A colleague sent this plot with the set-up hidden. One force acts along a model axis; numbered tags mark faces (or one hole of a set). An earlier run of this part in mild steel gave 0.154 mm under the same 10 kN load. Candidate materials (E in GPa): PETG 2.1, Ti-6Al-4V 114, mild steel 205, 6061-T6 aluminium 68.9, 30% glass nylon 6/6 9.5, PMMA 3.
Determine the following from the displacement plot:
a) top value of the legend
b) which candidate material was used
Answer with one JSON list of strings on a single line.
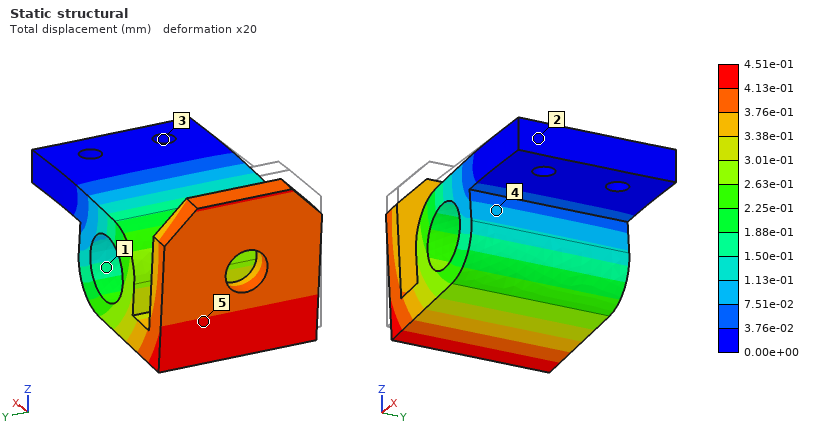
["4.51e-01 mm", "6061-T6 aluminium"]
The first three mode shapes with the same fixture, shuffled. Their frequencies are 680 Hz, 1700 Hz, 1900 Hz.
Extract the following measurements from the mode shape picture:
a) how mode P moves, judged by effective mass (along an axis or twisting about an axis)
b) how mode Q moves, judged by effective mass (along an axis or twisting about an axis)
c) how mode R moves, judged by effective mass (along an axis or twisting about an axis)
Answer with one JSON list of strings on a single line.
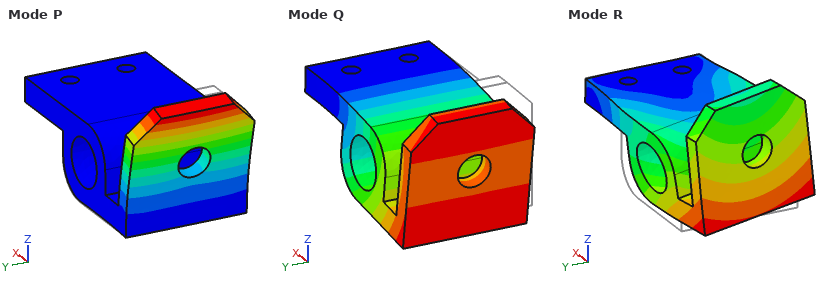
["along X", "along Z", "along Y"]
